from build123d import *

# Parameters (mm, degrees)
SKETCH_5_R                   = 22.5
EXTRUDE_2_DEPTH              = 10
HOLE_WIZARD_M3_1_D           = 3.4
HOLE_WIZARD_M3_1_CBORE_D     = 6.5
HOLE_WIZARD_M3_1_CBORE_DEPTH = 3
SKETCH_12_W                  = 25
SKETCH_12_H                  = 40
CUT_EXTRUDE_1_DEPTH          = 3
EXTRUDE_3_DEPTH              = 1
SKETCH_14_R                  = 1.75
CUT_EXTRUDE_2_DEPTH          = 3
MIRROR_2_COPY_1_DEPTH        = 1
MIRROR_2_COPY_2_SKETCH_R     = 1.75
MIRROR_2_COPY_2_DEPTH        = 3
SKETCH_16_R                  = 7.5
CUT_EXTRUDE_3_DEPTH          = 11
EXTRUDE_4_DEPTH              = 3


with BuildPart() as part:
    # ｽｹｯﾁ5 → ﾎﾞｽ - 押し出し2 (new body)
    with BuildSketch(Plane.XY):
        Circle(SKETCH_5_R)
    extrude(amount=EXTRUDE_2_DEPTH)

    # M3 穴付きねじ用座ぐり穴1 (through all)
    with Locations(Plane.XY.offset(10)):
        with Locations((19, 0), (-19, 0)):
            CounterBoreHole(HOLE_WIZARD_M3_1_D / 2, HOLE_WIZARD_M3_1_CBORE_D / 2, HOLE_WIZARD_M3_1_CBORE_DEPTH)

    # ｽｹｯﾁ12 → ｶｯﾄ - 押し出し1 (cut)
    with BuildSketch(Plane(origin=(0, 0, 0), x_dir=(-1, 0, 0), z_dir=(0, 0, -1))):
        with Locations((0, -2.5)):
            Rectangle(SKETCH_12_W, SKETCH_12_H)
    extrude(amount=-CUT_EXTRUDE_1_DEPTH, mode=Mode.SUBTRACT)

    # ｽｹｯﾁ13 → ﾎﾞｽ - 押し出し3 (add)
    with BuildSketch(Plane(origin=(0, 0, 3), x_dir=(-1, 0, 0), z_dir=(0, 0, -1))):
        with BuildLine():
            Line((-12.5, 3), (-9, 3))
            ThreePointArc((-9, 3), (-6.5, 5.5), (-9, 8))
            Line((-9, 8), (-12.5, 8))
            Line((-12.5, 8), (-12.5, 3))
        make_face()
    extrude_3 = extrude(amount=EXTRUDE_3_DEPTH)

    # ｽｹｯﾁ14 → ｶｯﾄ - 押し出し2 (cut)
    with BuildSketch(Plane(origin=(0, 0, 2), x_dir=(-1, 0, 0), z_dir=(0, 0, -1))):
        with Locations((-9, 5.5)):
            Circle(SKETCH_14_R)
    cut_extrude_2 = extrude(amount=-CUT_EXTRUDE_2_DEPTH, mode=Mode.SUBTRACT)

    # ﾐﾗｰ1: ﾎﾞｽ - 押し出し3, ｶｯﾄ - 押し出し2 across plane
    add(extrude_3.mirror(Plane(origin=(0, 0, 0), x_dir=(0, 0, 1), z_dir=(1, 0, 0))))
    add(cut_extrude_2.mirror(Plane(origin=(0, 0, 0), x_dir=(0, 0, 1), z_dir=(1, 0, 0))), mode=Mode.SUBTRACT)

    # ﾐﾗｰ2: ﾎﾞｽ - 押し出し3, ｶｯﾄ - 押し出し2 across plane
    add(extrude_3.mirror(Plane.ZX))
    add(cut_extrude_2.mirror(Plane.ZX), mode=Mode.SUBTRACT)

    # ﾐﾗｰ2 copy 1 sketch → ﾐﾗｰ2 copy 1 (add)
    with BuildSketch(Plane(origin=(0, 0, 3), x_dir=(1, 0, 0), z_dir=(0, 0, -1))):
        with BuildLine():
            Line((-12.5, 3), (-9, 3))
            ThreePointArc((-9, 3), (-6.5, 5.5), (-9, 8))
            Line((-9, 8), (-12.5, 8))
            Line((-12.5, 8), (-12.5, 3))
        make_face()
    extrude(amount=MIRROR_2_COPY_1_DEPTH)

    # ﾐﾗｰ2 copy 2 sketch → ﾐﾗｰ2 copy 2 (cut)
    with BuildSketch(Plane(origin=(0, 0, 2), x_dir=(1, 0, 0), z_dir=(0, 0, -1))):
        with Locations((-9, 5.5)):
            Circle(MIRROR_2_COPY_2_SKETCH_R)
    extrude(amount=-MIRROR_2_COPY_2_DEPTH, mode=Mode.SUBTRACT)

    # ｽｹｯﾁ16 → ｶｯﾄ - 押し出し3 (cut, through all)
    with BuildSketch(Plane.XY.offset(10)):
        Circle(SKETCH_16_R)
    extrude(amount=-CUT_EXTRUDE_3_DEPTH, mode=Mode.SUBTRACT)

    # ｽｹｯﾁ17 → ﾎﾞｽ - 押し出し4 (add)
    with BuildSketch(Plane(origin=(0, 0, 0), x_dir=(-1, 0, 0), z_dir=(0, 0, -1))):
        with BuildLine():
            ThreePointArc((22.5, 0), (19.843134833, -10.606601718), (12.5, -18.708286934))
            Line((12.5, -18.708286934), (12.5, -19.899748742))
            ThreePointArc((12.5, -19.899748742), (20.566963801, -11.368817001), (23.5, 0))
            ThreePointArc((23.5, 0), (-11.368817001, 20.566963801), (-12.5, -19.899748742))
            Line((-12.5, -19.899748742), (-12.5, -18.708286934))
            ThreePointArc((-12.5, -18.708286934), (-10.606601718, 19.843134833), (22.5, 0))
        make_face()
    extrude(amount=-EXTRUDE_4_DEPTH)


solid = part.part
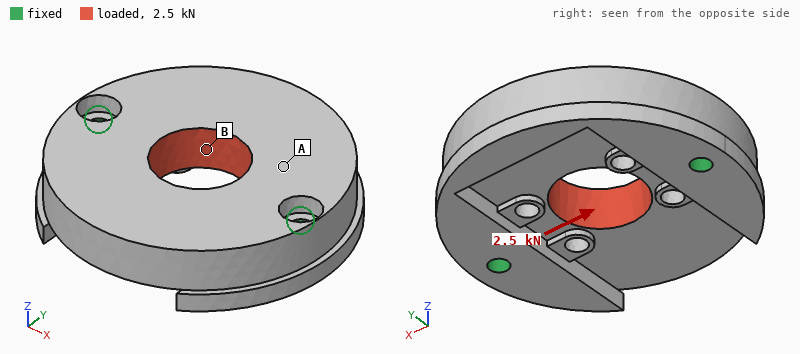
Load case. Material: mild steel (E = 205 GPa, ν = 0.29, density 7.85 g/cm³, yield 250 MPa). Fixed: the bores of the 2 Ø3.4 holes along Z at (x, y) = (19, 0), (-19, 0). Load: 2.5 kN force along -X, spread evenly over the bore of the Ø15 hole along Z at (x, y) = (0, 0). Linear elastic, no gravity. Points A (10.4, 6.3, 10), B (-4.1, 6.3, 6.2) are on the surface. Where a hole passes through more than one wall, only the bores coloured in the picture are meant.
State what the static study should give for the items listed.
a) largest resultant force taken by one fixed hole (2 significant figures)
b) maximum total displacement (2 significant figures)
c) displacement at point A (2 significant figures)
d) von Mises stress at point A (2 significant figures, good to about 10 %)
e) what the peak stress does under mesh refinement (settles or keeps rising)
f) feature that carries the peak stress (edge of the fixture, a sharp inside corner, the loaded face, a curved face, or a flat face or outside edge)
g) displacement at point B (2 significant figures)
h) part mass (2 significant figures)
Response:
1.3 kN
1.5 µm
1.1 µm
6.3 MPa
keeps rising
edge of the fixture
1.3 µm
92 g
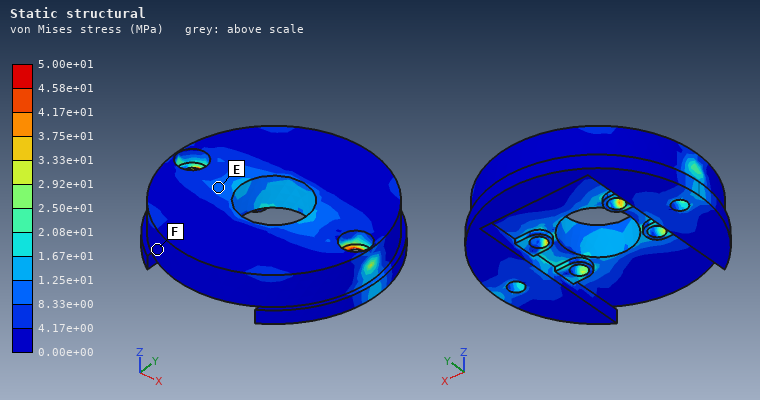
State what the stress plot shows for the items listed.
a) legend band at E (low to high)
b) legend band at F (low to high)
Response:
8.33e+00 to 1.25e+01 MPa
0.00e+00 to 4.17e+00 MPa
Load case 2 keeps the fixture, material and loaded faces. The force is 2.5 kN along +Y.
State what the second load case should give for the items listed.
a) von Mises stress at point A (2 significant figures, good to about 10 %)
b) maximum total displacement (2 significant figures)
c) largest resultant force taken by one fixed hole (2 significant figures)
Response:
8.8 MPa
4.5 µm
1.3 kN
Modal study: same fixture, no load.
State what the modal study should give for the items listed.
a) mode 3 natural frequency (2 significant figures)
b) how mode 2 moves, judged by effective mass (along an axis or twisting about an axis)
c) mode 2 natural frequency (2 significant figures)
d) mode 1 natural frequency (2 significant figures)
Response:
20 kHz
along Z
12 kHz
8400 Hz
